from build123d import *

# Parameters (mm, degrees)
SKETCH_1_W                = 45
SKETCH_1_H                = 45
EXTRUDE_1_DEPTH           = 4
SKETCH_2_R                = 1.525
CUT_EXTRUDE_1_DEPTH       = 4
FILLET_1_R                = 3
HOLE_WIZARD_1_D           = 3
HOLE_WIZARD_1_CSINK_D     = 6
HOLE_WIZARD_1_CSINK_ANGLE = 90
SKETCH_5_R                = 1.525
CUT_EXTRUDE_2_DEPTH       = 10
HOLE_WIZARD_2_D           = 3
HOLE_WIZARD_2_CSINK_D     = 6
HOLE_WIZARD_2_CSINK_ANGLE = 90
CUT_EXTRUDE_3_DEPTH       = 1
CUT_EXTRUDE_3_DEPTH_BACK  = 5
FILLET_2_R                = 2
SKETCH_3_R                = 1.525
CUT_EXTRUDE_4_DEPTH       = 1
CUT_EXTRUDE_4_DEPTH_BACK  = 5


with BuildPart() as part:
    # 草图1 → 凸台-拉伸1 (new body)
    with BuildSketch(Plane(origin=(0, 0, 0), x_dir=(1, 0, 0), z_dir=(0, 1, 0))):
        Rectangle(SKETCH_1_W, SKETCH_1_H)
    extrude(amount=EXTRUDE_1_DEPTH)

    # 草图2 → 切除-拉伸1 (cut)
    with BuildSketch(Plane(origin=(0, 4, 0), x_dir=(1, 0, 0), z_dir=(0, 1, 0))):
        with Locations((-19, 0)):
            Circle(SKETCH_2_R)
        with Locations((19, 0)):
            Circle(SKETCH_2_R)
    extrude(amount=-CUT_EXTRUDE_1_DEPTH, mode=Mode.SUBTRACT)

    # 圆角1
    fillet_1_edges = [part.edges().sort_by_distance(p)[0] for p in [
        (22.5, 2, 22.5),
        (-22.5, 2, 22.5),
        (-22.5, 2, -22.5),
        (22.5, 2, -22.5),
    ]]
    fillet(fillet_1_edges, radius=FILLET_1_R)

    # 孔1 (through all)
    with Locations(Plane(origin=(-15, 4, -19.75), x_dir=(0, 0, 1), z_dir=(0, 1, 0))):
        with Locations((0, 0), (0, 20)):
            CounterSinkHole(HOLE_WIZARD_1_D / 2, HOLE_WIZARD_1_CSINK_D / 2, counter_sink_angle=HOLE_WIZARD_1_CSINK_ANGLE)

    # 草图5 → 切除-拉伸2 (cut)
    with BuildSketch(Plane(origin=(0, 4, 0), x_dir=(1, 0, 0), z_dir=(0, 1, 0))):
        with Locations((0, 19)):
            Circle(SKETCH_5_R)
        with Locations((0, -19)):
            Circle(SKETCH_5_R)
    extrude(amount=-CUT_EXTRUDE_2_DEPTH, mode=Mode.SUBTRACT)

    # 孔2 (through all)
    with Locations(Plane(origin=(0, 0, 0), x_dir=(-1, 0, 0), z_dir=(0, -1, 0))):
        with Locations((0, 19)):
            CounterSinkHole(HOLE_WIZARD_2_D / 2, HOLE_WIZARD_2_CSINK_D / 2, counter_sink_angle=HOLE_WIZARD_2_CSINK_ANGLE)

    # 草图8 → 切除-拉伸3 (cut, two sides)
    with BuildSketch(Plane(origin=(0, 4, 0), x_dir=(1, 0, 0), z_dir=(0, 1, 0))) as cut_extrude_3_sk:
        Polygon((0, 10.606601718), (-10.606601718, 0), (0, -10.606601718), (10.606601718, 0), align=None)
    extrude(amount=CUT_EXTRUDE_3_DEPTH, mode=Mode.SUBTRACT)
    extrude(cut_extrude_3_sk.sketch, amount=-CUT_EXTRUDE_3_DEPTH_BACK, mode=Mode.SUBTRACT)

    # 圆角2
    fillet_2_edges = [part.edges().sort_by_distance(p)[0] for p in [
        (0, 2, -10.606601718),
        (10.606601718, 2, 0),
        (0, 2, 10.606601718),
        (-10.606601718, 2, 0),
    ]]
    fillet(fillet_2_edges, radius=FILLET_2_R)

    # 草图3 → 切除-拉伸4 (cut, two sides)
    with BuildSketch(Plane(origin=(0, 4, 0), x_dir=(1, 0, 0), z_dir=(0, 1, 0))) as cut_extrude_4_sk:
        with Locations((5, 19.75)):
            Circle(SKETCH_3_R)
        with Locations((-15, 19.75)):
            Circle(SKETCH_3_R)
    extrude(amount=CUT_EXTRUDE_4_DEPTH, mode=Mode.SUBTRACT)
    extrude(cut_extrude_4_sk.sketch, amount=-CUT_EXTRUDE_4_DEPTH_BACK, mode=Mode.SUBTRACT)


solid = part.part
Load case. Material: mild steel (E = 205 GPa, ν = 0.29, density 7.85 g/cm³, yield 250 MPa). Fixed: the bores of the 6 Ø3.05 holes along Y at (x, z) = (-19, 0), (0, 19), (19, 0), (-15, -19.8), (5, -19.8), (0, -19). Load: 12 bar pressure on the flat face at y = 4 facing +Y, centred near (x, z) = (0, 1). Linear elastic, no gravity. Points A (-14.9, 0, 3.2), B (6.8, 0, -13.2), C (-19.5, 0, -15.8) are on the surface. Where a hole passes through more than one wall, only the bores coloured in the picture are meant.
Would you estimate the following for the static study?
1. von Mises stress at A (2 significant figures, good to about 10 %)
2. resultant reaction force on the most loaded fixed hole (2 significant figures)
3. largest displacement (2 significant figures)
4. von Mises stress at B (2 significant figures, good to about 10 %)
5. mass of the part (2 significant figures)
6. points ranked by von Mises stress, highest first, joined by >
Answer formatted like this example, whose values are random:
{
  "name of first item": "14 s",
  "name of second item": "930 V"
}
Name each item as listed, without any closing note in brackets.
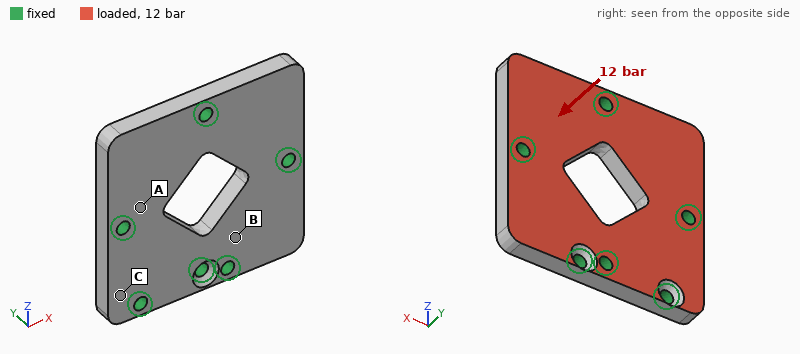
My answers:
{
  "von Mises stress at A": "21 MPa",
  "resultant reaction force on the most loaded fixed hole": "540 N",
  "largest displacement": "10 µm",
  "von Mises stress at B": "14 MPa",
  "mass of the part": "55 g",
  "points ranked by von Mises stress, highest first, joined by >": "A > B > C"
}
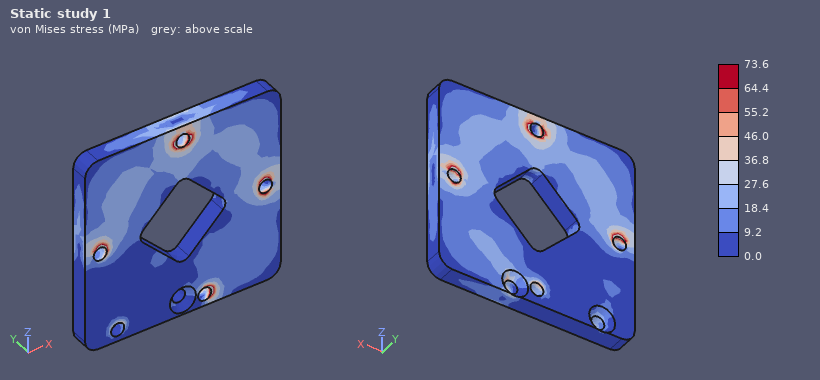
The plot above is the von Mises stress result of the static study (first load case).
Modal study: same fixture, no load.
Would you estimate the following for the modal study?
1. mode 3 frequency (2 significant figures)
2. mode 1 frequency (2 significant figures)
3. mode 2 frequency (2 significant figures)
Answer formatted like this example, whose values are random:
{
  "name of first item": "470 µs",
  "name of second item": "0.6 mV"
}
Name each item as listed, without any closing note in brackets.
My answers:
{
  "mode 3 frequency": "15 kHz",
  "mode 1 frequency": "12 kHz",
  "mode 2 frequency": "13 kHz"
}
